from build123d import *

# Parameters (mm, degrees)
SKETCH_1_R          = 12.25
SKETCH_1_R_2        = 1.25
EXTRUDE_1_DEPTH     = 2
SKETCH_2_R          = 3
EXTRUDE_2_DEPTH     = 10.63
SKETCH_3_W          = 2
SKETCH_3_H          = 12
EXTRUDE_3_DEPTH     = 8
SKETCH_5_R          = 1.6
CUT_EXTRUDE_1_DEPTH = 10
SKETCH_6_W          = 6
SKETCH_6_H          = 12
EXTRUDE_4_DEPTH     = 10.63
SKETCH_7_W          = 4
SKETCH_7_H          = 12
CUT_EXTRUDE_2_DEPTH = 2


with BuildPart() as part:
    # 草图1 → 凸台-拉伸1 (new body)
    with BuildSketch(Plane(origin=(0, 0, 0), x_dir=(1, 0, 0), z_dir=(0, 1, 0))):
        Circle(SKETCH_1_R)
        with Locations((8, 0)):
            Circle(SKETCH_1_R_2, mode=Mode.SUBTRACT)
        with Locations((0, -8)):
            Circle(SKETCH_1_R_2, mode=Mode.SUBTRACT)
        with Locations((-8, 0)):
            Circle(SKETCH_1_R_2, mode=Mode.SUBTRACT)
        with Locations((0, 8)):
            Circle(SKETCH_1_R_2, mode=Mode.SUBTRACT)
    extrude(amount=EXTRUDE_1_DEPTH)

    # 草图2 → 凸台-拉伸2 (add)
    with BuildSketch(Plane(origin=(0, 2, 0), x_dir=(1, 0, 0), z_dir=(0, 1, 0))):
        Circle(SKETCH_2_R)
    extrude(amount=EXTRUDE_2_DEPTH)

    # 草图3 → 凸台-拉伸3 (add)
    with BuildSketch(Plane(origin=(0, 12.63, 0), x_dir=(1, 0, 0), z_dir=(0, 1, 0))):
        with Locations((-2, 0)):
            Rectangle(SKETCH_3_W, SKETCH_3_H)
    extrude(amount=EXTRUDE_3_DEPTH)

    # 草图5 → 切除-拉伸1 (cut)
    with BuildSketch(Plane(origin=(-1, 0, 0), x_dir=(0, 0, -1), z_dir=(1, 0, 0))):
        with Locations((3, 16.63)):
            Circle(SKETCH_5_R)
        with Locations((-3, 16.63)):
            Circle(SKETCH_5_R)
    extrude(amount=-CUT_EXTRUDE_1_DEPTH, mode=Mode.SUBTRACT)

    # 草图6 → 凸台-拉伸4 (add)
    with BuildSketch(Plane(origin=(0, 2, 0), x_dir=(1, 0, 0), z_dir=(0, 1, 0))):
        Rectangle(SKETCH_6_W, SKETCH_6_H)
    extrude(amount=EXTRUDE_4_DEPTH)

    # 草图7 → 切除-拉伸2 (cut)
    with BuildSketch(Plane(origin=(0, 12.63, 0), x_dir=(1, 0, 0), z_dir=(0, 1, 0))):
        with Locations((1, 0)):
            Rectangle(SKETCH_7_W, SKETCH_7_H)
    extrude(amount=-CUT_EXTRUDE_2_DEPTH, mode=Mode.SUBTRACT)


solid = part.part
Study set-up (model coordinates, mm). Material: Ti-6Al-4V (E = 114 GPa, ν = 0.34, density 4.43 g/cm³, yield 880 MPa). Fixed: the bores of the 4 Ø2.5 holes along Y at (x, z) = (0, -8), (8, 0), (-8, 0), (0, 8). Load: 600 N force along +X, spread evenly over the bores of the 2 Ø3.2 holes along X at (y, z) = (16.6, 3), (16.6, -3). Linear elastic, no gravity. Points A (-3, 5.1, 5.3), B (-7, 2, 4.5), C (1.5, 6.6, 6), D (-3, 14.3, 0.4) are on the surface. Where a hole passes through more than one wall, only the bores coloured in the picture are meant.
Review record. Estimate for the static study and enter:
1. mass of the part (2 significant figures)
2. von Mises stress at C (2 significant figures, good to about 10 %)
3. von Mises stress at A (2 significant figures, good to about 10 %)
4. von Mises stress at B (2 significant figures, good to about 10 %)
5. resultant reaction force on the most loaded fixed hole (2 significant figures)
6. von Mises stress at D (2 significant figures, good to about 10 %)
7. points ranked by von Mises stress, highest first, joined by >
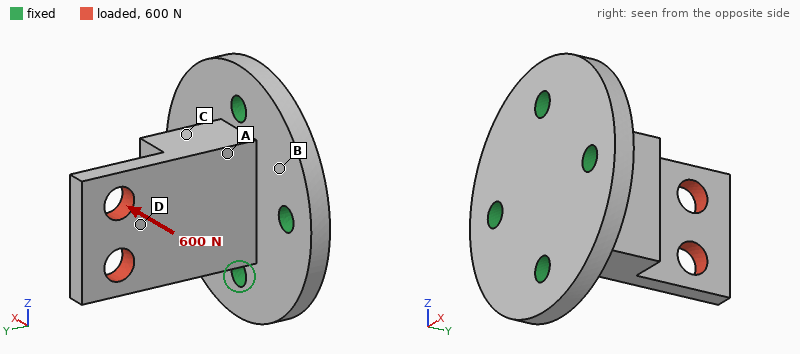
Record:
7.7 g
59 MPa
100 MPa
29 MPa
590 N
190 MPa
D > A > C > B
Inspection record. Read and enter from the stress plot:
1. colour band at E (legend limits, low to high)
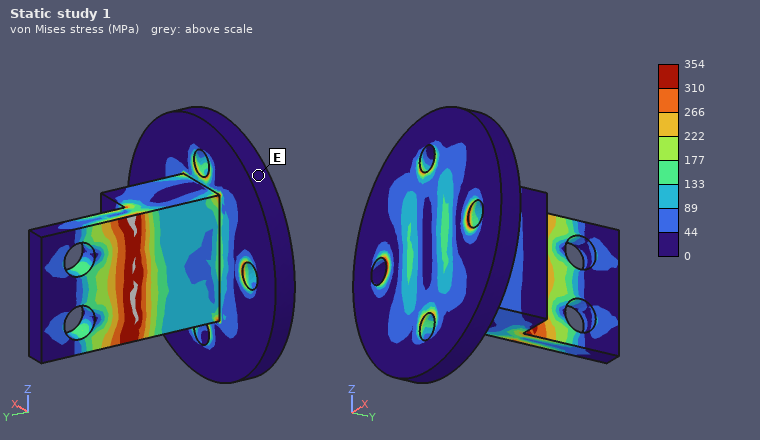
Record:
0 to 44 MPa
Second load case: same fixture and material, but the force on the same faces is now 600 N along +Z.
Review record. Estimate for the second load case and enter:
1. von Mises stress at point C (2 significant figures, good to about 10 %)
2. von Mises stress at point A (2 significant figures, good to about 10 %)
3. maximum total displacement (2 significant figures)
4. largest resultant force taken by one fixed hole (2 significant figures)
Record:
33 MPa
61 MPa
37 µm
720 N
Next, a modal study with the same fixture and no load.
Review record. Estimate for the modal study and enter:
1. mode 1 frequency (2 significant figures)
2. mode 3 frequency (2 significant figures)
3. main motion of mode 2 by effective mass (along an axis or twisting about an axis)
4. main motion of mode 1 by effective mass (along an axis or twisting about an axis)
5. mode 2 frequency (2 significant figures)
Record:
11 kHz
25 kHz
along Z
along X
23 kHz
